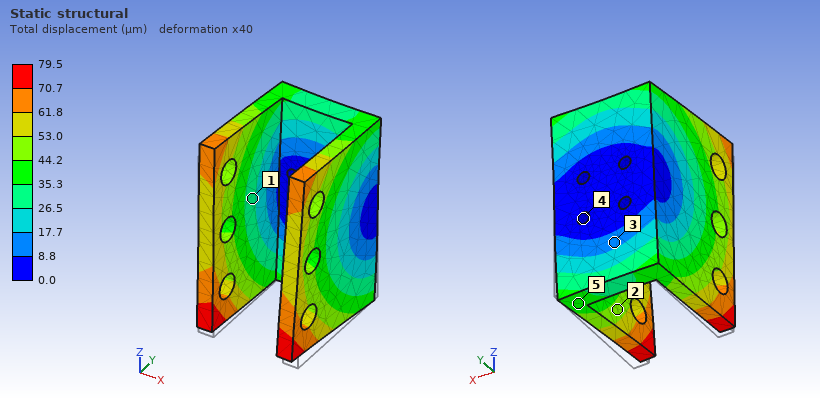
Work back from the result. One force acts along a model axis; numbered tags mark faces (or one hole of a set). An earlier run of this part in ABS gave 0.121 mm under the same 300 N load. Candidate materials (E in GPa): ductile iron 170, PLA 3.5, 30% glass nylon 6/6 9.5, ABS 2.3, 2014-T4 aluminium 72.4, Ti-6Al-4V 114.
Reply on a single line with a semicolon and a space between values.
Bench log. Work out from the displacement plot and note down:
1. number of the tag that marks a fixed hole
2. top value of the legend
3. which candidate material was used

4; 79.5 µm; PLA
